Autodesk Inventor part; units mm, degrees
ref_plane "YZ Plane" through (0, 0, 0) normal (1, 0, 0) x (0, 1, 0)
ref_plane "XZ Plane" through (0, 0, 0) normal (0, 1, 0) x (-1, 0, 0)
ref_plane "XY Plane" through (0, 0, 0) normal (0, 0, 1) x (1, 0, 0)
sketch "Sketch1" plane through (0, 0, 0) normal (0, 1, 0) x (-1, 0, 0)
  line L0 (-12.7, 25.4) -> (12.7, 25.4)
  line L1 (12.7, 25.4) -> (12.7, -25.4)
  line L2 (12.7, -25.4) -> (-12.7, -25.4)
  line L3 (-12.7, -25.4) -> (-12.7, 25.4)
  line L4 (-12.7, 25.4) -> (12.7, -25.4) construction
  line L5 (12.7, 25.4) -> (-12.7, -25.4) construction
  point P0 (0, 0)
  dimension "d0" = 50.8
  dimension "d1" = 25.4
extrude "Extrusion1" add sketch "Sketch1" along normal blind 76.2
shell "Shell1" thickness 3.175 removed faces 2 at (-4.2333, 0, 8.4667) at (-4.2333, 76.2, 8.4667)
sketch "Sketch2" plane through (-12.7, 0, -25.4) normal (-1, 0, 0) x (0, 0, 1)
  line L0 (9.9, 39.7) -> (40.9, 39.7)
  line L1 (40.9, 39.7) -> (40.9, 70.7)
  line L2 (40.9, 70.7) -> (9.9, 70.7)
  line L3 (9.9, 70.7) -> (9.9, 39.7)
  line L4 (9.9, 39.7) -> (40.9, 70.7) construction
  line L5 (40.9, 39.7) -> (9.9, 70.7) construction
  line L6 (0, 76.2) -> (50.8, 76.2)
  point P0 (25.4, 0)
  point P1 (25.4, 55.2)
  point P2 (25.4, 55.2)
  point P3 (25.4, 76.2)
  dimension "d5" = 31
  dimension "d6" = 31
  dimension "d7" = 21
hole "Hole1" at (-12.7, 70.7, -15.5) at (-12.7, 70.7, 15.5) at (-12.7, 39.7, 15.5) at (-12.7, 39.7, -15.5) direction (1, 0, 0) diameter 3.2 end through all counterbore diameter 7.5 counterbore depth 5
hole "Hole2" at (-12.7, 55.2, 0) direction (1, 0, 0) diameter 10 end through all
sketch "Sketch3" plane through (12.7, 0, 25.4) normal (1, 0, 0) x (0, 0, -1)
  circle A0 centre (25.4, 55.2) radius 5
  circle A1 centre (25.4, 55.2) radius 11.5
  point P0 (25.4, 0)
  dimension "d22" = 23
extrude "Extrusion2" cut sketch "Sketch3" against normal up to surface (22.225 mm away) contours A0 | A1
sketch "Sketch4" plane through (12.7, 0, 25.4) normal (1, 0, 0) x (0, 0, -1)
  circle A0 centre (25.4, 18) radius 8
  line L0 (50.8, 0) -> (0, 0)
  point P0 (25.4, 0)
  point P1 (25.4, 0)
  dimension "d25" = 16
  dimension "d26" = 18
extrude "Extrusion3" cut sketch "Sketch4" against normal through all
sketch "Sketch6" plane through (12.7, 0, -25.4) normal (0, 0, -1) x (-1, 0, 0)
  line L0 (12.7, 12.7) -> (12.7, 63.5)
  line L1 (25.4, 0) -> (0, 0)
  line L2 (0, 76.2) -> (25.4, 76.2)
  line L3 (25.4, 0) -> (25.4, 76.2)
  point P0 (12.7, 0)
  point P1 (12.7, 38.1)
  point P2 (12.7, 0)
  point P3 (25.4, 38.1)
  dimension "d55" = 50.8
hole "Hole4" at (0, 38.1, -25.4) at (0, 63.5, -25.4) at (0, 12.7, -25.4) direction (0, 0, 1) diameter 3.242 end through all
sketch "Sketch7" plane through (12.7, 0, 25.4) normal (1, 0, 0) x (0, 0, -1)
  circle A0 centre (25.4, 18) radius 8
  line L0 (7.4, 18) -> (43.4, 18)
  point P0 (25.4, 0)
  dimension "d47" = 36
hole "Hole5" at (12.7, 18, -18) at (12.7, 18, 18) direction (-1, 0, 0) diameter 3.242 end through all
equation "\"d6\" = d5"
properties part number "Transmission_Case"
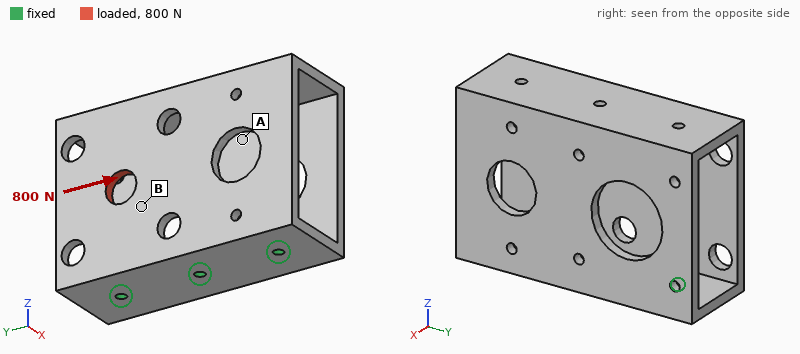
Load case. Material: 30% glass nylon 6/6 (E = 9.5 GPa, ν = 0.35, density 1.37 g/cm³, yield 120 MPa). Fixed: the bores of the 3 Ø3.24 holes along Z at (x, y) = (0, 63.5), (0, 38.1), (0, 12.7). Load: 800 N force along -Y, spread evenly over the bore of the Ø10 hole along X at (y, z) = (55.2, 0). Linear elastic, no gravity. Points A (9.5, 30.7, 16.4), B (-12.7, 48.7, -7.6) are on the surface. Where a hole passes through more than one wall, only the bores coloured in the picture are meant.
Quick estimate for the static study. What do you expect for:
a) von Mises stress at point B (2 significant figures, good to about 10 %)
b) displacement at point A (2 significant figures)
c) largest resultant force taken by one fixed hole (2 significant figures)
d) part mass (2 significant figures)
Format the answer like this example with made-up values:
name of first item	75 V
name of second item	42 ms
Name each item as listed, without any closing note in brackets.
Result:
von Mises stress at point B	10 MPa
displacement at point A	0.12 mm
largest resultant force taken by one fixed hole	480 N
part mass	41 g
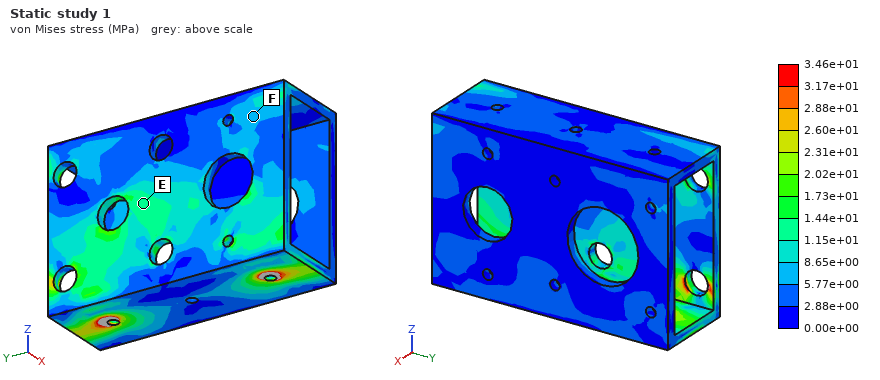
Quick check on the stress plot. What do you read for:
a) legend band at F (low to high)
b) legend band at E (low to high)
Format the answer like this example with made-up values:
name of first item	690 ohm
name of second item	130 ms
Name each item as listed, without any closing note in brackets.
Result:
legend band at F	5.77e+00 to 8.65e+00 MPa
legend band at E	1.15e+01 to 1.44e+01 MPa
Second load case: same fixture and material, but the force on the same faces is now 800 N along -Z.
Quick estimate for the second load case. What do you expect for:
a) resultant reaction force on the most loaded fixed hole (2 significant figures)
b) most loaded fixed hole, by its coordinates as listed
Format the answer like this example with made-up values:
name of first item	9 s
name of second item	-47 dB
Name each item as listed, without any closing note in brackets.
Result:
resultant reaction force on the most loaded fixed hole	520 N
most loaded fixed hole, by its coordinates as listed	(0, 63.5)
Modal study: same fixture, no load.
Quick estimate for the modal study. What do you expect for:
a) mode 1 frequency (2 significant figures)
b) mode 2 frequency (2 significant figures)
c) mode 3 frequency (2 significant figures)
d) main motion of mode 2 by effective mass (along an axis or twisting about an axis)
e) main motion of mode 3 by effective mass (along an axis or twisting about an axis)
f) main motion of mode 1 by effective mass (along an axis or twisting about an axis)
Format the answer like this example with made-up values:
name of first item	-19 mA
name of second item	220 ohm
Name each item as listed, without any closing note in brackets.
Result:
mode 1 frequency	420 Hz
mode 2 frequency	1400 Hz
mode 3 frequency	1500 Hz
main motion of mode 2 by effective mass	twisting about Z
main motion of mode 3 by effective mass	along Y
main motion of mode 1 by effective mass	along X
